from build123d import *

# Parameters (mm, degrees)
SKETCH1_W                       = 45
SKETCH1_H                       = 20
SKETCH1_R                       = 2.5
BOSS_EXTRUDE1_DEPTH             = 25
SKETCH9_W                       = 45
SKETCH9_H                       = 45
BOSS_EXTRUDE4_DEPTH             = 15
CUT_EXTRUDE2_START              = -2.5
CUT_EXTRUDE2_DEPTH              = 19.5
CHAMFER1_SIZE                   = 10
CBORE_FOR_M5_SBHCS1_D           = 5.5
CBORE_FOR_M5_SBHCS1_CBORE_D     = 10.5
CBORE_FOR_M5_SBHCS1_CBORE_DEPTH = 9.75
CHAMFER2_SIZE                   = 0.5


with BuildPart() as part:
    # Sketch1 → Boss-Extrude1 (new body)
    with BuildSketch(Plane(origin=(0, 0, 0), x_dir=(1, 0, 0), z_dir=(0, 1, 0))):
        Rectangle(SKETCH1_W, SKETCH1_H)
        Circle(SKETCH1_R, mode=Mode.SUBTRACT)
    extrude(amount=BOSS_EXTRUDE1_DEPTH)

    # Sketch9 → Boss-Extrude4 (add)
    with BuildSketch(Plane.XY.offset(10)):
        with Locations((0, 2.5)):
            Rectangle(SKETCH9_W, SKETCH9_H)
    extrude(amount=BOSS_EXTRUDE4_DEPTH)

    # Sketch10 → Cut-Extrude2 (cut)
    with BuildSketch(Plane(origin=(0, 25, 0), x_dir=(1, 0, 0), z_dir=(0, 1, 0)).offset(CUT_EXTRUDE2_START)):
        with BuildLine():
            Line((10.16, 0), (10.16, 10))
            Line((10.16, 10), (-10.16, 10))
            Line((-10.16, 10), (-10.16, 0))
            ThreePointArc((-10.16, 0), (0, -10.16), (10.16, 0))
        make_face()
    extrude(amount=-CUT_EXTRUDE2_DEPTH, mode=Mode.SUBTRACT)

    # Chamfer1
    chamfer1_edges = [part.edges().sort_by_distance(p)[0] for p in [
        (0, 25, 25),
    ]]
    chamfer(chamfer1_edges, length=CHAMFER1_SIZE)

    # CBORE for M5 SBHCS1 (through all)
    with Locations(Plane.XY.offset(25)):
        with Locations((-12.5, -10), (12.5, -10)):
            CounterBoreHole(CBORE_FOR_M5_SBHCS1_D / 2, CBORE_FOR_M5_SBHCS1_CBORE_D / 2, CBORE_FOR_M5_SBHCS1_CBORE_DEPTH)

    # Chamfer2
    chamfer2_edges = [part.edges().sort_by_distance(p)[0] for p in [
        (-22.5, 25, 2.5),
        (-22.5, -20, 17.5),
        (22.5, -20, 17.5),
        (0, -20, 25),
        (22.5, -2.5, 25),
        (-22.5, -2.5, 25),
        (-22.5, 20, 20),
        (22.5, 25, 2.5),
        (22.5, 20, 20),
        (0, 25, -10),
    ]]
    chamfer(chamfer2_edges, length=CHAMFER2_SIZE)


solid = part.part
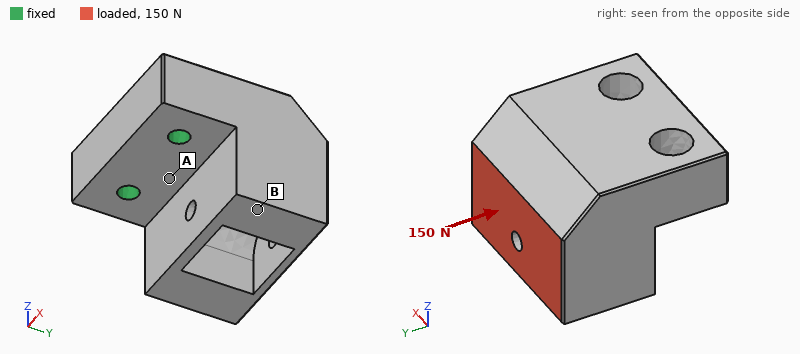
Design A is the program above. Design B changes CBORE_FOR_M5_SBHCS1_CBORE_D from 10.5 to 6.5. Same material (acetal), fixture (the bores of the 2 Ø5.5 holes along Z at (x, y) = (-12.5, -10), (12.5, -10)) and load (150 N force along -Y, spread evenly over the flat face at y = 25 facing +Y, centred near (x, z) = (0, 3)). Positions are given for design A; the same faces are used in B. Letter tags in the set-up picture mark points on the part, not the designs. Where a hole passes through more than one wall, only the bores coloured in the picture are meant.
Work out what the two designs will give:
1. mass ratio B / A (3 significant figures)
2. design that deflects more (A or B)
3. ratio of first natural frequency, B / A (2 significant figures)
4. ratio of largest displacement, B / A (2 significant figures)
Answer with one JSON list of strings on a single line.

["1.03", "A", "1.1", "0.91"]
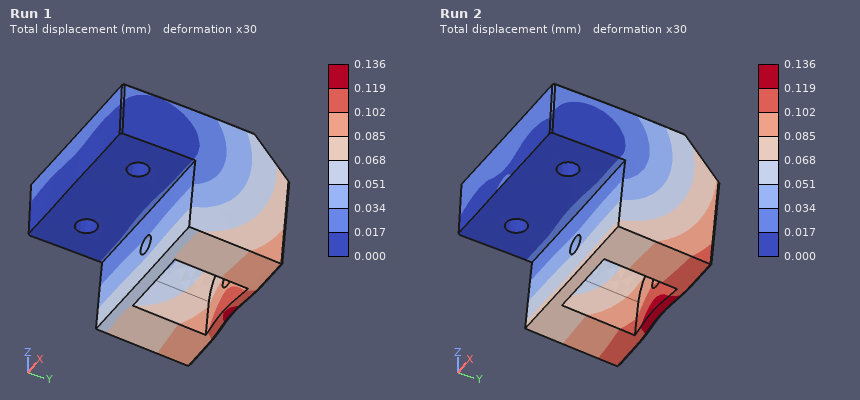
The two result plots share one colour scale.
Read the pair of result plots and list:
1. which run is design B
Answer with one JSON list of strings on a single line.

["Run 1"]
